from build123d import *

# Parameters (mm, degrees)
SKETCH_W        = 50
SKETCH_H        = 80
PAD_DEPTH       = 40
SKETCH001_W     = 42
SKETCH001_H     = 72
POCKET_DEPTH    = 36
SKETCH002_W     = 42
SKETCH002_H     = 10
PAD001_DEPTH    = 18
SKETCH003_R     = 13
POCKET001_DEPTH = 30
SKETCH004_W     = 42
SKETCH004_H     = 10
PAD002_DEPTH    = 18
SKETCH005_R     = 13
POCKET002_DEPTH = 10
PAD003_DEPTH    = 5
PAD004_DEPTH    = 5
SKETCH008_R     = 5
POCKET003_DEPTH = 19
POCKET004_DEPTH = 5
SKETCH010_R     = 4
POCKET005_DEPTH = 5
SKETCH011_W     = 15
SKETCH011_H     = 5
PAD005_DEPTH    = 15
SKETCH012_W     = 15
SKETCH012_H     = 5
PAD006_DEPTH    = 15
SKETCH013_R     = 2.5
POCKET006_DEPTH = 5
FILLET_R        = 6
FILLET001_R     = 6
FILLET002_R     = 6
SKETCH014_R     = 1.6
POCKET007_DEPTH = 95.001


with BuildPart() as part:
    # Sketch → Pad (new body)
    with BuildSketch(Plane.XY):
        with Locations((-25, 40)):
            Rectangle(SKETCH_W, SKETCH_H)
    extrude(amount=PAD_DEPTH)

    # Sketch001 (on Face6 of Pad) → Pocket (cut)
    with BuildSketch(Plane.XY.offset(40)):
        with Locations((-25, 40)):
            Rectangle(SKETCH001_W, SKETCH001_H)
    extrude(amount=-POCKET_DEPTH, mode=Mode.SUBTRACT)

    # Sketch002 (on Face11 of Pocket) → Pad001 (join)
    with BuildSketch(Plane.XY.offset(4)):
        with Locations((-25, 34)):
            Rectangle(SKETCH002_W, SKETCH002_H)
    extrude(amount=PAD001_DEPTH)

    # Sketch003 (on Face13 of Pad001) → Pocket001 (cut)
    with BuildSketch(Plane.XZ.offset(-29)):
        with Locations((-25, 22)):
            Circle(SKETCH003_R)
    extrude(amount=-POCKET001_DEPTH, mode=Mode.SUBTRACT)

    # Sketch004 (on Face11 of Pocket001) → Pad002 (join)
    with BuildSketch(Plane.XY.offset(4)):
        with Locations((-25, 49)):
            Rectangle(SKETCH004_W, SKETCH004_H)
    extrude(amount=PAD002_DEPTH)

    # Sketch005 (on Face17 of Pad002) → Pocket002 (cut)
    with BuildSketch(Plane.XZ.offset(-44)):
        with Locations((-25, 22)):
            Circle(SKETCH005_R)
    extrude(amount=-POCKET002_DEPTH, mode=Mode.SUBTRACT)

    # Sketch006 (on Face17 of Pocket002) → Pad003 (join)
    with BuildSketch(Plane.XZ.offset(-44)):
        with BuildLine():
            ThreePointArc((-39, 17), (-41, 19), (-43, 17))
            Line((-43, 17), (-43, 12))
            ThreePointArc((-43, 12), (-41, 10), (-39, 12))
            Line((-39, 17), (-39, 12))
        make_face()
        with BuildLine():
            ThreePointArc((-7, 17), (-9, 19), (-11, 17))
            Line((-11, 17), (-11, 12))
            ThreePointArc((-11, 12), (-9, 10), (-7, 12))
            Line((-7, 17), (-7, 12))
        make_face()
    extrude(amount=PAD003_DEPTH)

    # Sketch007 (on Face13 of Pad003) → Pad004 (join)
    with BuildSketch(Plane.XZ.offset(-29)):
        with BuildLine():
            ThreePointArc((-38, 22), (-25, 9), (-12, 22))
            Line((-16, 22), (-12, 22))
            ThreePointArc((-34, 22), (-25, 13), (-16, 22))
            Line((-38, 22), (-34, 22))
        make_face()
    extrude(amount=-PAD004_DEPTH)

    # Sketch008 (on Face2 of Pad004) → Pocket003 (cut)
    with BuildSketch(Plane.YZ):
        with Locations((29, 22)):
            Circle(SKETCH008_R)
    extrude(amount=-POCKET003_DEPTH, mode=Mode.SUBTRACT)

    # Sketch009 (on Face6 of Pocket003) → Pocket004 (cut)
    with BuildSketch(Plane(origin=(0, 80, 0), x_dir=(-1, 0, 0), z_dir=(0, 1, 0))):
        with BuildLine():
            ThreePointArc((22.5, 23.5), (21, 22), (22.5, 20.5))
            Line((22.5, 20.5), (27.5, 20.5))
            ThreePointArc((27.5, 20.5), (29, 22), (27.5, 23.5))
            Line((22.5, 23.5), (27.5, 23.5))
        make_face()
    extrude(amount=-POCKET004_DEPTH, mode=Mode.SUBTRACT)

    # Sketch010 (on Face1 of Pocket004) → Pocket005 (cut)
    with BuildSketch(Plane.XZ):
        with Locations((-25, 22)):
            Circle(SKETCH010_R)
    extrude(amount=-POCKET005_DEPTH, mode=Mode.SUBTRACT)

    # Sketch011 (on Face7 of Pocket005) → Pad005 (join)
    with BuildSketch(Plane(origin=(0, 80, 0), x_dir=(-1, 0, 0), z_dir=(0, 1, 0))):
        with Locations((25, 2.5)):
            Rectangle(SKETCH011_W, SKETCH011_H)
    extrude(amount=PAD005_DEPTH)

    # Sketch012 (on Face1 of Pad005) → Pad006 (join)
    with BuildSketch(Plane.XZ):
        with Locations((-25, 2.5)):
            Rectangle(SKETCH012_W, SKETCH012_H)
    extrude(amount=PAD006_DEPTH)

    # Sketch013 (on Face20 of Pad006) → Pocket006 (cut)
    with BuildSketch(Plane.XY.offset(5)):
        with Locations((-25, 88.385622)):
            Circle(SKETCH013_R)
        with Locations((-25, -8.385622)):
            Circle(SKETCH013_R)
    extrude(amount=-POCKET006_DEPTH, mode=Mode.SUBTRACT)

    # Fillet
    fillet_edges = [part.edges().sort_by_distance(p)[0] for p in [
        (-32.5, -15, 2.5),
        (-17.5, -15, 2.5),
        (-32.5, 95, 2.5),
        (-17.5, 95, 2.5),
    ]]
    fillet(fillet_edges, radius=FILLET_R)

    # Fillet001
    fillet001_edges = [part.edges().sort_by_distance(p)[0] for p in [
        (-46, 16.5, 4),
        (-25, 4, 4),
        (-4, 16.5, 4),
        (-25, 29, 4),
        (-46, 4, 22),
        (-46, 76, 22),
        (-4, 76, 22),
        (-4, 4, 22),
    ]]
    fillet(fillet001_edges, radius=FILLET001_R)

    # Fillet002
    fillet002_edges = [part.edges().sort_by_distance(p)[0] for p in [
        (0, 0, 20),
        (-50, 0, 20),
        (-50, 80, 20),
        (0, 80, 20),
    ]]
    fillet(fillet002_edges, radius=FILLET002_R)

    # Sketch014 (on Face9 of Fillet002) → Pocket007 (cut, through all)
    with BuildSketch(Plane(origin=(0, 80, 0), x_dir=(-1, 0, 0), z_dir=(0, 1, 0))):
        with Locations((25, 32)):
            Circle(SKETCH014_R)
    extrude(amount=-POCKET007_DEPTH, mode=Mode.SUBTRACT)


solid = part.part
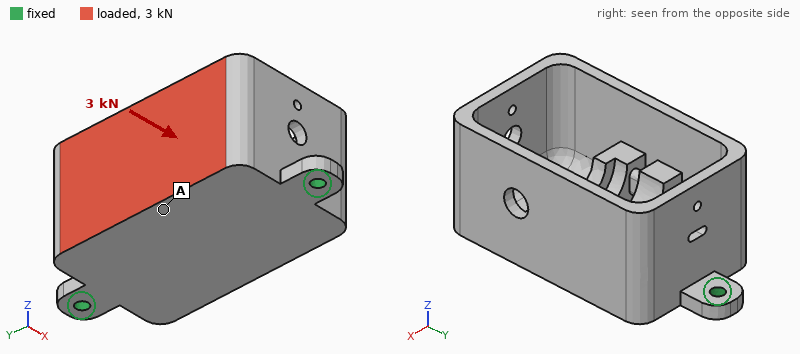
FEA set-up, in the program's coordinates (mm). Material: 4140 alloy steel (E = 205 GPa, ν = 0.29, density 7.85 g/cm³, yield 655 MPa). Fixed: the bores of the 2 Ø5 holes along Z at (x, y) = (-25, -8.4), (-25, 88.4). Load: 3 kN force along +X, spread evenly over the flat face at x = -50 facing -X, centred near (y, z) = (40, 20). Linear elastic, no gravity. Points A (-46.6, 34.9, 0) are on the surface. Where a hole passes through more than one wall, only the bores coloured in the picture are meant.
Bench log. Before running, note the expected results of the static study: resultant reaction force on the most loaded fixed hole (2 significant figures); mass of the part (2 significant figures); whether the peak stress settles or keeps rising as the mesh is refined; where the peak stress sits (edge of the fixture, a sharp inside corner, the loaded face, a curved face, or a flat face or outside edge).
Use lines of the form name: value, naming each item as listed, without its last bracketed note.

resultant reaction force on the most loaded fixed hole: 1.5 kN
mass of the part: 500 g
whether the peak stress settles or keeps rising as the mesh is refined: keeps rising
where the peak stress sits: edge of the fixture
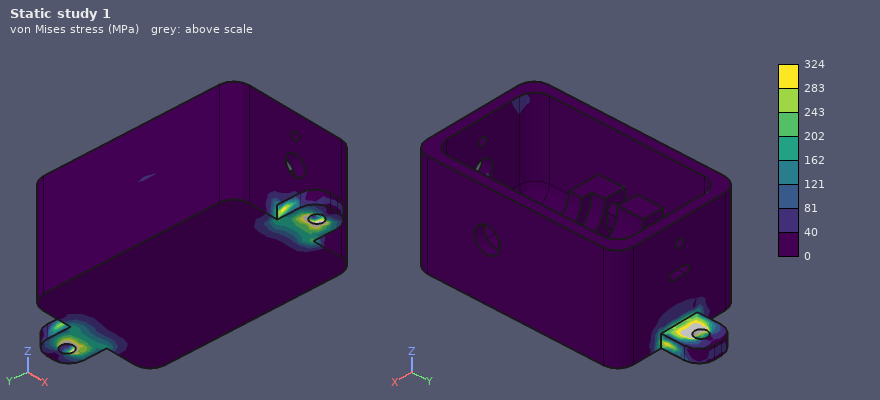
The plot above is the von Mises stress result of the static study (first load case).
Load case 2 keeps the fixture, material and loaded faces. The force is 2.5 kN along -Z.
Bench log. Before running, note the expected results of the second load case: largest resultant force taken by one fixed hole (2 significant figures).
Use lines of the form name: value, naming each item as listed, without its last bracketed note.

largest resultant force taken by one fixed hole: 1.3 kN
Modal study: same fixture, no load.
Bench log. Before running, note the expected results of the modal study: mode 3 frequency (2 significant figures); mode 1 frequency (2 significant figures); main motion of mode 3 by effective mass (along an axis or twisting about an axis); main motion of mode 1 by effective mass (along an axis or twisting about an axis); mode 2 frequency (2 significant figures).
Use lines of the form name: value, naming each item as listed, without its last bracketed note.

mode 3 frequency: 3600 Hz
mode 1 frequency: 980 Hz
main motion of mode 3 by effective mass: along Z
main motion of mode 1 by effective mass: along X
mode 2 frequency: 3500 Hz
